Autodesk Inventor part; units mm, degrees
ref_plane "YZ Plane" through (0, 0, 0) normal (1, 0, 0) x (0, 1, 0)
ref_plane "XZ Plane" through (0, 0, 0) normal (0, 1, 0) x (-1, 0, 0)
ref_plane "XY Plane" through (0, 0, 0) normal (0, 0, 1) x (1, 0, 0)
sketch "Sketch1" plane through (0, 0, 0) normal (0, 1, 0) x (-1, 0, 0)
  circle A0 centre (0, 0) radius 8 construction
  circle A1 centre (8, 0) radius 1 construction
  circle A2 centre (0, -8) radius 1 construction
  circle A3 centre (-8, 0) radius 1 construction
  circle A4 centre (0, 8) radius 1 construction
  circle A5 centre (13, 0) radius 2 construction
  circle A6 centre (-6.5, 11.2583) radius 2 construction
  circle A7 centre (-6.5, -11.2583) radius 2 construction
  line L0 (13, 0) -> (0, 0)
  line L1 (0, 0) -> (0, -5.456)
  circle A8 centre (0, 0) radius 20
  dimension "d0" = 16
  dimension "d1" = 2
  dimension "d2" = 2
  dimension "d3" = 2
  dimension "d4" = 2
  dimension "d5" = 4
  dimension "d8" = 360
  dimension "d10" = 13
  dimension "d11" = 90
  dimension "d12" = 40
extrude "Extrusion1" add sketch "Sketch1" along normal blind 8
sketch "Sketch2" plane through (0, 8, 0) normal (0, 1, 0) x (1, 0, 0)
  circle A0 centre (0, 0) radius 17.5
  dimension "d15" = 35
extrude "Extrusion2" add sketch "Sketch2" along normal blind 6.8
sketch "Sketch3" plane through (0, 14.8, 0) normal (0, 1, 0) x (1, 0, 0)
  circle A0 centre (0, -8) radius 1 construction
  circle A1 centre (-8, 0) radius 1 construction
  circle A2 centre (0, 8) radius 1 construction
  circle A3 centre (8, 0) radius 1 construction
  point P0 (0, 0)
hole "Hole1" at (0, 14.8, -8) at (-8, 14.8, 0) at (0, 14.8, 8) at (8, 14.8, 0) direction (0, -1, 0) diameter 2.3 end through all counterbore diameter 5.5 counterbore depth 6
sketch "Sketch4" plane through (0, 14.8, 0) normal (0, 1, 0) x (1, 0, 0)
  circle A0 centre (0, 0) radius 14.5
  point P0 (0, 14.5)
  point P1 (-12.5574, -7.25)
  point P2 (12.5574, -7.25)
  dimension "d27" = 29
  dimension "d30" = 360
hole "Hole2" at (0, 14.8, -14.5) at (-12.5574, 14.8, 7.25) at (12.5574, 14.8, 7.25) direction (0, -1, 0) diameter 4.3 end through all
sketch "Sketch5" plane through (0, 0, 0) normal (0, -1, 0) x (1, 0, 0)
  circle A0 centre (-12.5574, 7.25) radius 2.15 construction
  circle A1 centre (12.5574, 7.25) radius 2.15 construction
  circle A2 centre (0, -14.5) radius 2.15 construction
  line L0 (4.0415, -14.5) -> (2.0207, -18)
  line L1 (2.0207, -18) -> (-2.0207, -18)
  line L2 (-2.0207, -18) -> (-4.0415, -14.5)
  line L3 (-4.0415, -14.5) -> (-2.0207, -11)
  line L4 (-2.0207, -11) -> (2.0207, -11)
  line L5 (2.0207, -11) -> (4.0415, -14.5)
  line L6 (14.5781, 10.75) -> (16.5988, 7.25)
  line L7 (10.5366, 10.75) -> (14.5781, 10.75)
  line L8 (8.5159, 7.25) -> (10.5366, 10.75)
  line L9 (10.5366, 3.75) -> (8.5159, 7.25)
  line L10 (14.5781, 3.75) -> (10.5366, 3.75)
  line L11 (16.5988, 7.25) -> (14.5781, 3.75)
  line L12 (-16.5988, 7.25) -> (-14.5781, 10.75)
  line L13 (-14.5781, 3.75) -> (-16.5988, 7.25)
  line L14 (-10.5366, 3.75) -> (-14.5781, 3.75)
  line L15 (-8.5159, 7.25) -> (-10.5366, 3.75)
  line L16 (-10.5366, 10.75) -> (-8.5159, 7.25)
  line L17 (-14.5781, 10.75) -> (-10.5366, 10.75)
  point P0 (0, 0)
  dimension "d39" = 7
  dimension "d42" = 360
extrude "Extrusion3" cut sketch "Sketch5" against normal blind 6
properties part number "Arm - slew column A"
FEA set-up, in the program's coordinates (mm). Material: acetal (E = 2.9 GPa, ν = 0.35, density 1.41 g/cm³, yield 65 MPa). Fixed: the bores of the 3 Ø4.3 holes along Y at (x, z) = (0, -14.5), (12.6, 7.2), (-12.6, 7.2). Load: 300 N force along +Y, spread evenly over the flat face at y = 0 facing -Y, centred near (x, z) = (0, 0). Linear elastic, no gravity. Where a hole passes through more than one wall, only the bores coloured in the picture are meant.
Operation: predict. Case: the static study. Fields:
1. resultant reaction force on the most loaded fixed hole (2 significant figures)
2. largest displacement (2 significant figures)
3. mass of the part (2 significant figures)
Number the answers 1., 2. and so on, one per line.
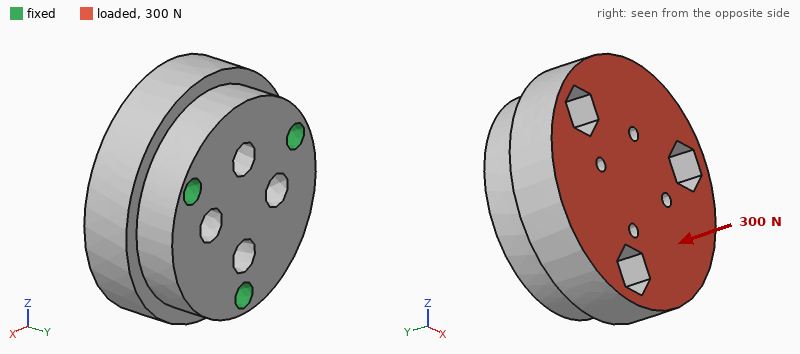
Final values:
1. 100 N
2. 6.9 µm
3. 21 g
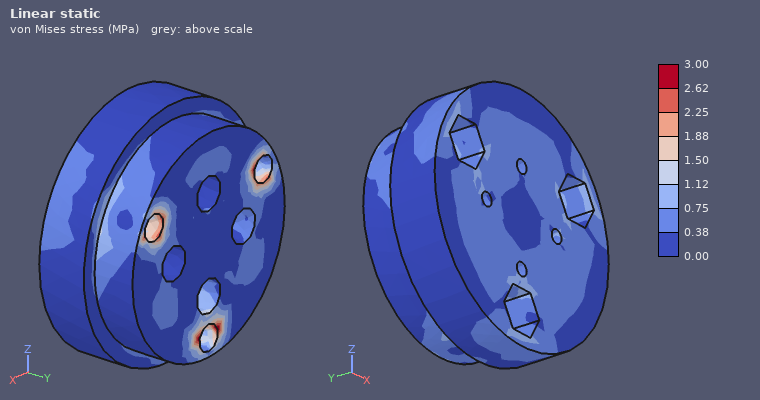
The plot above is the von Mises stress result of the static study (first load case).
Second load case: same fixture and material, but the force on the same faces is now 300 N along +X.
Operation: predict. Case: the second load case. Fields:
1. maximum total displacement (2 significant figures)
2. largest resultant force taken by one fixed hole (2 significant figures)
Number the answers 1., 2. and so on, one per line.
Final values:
1. 16 µm
2. 140 N
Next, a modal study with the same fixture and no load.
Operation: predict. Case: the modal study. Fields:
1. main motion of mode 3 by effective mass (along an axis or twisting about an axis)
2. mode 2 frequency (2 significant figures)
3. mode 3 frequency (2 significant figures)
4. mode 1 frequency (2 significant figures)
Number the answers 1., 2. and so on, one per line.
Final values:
1. along Y
2. 8000 Hz
3. 9800 Hz
4. 8000 Hz
